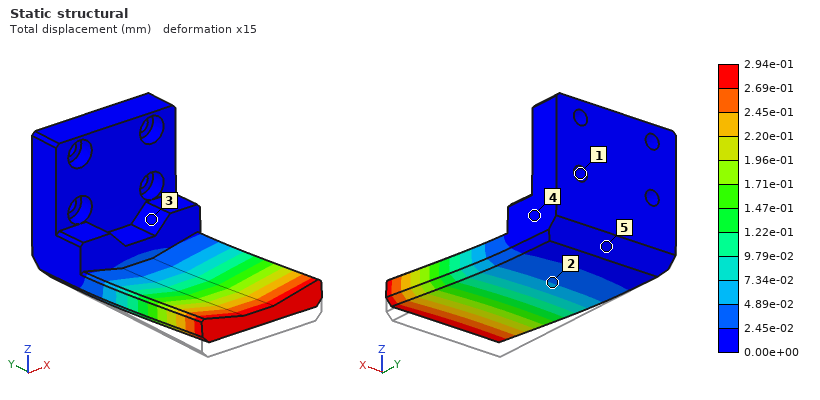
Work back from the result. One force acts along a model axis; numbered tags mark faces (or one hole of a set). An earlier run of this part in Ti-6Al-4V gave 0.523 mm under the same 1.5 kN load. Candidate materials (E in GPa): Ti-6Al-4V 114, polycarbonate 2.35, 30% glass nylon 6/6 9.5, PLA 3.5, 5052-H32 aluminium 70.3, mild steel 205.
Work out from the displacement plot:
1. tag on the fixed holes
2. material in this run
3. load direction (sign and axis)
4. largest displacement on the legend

1
mild steel
+Z
2.94e-01 mm
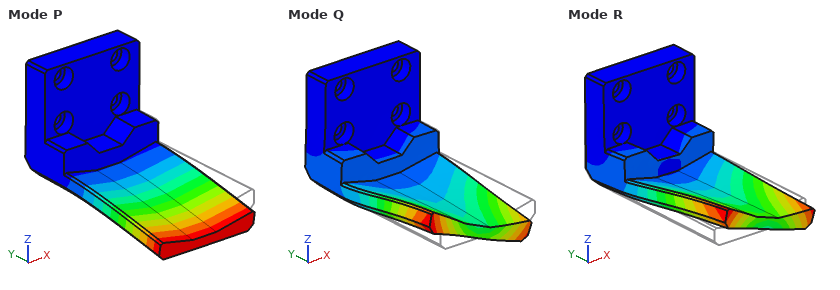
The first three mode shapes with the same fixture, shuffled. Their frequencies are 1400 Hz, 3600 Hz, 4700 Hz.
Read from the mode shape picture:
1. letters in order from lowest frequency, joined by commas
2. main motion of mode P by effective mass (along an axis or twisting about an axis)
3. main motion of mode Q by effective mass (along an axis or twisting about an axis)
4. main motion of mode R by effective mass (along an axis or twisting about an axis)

P, R, Q
along Z
along X
along X
